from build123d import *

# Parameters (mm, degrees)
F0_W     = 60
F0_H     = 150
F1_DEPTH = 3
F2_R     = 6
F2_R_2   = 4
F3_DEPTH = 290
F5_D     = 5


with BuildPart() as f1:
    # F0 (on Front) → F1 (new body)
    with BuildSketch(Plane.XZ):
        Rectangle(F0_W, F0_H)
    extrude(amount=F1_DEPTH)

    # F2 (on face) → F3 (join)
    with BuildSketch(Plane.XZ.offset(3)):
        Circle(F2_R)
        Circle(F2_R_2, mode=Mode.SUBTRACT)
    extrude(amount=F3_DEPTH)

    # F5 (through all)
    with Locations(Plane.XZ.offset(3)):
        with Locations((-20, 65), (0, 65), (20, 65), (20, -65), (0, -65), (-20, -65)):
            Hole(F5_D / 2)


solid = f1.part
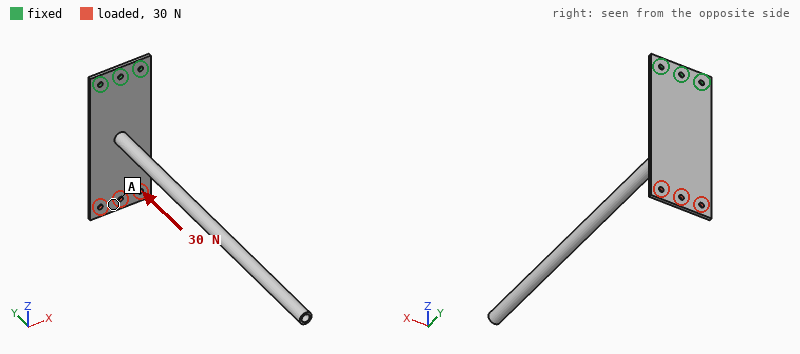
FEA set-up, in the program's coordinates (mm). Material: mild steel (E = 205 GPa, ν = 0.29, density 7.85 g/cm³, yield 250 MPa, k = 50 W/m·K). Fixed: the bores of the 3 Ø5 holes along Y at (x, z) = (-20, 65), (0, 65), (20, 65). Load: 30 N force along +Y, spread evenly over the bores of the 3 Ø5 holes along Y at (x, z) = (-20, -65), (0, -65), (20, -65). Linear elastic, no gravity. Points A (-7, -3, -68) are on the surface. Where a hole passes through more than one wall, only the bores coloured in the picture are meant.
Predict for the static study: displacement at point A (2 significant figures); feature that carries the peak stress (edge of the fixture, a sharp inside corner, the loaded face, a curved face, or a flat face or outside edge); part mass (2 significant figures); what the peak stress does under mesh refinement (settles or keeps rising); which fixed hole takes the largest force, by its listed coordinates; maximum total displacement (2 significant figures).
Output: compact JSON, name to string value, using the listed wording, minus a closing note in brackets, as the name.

{"displacement at point A": "0.77 mm", "feature that carries the peak stress": "edge of the fixture", "part mass": "350 g", "what the peak stress does under mesh refinement": "keeps rising", "which fixed hole takes the largest force, by its listed coordinates": "(0, 65)", "maximum total displacement": "1.9 mm"}
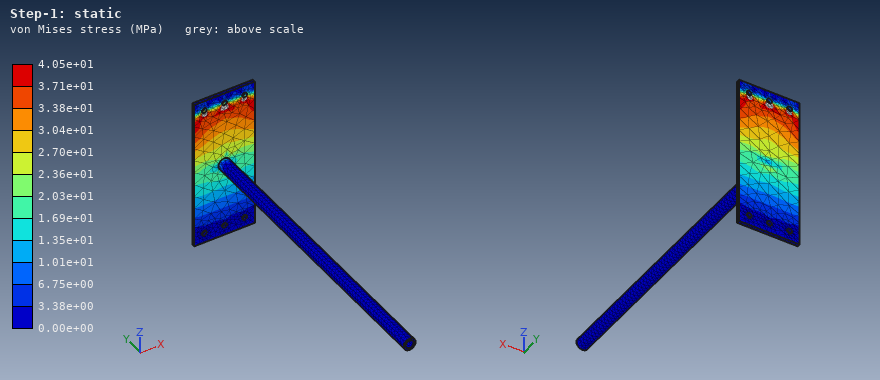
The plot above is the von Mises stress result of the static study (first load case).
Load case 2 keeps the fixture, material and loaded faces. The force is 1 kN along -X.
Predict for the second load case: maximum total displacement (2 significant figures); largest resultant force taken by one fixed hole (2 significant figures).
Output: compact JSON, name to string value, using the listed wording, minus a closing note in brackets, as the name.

{"maximum total displacement": "95 µm", "largest resultant force taken by one fixed hole": "3.1 kN"}
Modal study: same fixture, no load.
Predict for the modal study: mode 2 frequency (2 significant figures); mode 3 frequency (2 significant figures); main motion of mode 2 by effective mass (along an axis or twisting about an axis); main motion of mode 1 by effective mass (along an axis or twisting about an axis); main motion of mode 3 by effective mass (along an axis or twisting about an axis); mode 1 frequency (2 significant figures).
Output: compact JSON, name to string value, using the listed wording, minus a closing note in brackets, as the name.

{"mode 2 frequency": "63 Hz", "mode 3 frequency": "230 Hz", "main motion of mode 2 by effective mass": "along X", "main motion of mode 1 by effective mass": "along Z", "main motion of mode 3 by effective mass": "along Y", "mode 1 frequency": "46 Hz"}
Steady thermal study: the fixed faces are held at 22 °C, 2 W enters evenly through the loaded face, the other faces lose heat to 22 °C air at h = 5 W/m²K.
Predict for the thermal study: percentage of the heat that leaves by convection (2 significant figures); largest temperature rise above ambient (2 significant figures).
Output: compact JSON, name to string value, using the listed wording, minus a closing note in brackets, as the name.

{"percentage of the heat that leaves by convection": "51 %", "largest temperature rise above ambient": "20 K"}
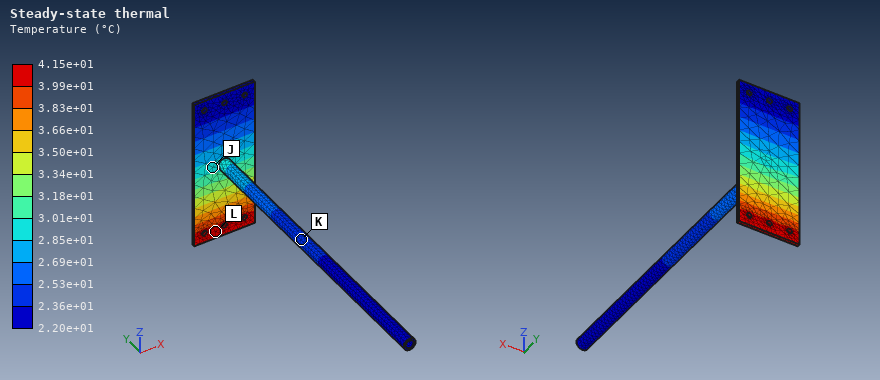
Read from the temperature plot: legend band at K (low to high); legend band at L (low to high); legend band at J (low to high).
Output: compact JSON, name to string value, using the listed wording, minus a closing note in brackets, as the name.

{"legend band at K": "2.36e+01 to 2.53e+01 °C", "legend band at L": "3.99e+01 to 4.15e+01 °C", "legend band at J": "2.85e+01 to 3.01e+01 °C"}
